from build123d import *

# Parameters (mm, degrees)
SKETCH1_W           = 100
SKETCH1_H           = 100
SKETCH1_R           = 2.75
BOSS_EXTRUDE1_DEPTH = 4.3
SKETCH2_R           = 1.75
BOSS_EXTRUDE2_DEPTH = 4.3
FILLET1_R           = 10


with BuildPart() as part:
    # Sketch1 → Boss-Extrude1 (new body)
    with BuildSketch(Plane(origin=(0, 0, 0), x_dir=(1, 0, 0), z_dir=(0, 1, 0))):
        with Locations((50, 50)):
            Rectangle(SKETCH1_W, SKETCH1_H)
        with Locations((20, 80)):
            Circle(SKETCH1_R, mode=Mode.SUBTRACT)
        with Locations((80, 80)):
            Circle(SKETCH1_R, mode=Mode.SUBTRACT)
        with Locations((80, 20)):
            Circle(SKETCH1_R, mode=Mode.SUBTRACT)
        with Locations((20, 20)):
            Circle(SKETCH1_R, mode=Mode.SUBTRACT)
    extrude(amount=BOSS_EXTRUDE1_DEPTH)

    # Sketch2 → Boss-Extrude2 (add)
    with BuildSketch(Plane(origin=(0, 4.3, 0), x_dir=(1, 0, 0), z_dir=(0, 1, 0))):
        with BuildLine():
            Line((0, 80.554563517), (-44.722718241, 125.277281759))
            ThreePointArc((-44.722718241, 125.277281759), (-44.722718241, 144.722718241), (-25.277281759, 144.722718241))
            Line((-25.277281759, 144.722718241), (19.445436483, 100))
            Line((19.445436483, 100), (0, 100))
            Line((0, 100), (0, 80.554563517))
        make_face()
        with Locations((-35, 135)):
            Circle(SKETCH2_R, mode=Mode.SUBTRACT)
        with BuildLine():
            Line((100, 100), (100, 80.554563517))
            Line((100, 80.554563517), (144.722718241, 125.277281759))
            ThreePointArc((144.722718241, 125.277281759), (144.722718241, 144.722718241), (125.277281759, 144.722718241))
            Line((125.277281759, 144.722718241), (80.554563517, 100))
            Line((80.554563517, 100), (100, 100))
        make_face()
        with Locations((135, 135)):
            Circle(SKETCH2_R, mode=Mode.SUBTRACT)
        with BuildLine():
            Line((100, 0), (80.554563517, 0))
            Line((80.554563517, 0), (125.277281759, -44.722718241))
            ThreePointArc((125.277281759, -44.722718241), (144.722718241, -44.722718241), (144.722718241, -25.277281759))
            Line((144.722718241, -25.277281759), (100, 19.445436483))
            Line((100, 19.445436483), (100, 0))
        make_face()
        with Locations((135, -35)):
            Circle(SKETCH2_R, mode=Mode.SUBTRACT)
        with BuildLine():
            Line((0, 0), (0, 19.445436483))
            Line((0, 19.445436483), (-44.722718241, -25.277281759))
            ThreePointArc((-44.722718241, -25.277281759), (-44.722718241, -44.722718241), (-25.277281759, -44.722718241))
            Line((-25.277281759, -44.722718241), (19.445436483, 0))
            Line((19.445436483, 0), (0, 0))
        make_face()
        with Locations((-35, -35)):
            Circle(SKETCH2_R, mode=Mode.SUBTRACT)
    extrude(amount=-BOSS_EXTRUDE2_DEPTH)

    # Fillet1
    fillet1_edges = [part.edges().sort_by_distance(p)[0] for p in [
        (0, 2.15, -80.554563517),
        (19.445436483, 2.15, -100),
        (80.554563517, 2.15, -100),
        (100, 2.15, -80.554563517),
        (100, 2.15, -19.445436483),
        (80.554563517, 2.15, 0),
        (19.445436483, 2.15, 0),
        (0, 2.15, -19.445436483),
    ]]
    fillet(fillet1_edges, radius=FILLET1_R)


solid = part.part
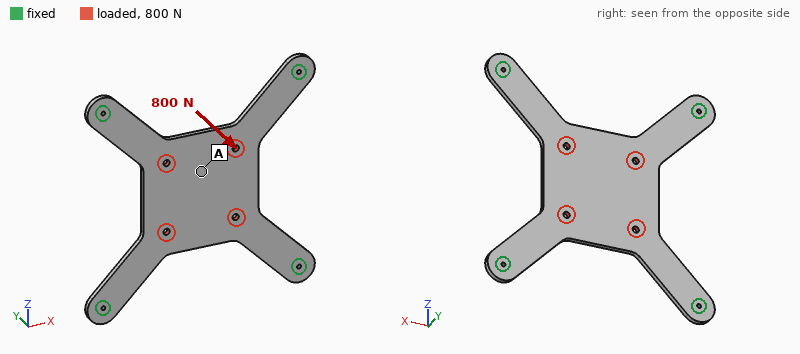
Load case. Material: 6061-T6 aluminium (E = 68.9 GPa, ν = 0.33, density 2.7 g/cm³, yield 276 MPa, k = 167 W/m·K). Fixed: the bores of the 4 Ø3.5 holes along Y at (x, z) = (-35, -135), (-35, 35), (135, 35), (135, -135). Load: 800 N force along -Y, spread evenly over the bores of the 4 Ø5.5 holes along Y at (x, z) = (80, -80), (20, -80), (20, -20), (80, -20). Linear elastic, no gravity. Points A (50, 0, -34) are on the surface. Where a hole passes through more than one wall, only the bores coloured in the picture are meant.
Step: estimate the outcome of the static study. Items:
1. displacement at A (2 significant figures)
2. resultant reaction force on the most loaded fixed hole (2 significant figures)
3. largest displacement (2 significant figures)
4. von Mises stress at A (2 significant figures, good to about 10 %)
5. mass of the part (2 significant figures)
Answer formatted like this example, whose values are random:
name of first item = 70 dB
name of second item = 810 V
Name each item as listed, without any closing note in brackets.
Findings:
displacement at A = 0.99 mm
resultant reaction force on the most loaded fixed hole = 200 N
largest displacement = 1.0 mm
von Mises stress at A = 29 MPa
mass of the part = 200 g
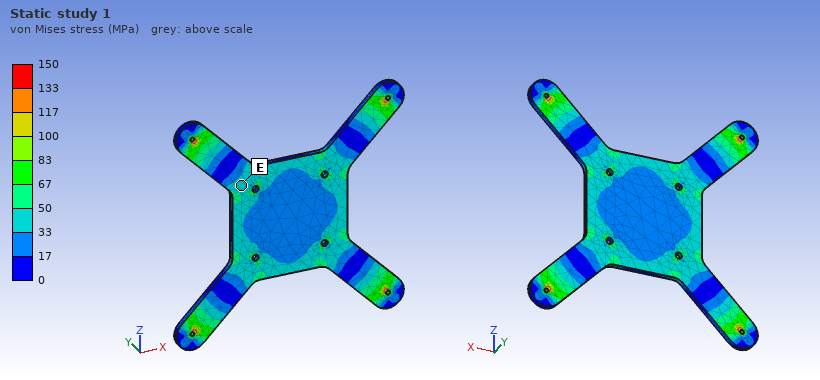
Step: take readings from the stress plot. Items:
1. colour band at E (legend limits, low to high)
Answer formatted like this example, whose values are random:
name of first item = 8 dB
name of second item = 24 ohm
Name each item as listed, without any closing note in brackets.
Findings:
colour band at E = 33 to 50 MPa
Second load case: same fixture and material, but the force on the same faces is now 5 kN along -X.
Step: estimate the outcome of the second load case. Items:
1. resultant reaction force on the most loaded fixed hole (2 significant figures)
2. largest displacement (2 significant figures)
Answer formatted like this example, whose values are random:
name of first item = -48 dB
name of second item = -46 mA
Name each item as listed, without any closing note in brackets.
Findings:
resultant reaction force on the most loaded fixed hole = 1.7 kN
largest displacement = 29 µm
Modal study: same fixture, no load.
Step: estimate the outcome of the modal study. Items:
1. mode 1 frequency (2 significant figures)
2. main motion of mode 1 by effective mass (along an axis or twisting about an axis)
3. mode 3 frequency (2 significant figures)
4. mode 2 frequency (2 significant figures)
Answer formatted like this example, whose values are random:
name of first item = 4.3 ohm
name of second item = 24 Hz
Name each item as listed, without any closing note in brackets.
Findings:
mode 1 frequency = 420 Hz
main motion of mode 1 by effective mass = along Y
mode 3 frequency = 980 Hz
mode 2 frequency = 980 Hz
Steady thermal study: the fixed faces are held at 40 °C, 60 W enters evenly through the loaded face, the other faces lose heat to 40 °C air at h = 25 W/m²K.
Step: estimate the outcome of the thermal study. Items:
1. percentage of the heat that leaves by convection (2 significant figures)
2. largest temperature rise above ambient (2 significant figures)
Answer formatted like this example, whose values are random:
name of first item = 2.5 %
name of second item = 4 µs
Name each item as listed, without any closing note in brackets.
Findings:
percentage of the heat that leaves by convection = 41 %
largest temperature rise above ambient = 42 K
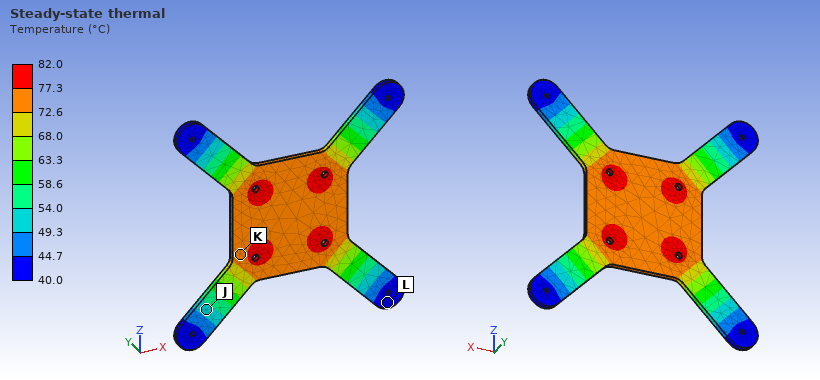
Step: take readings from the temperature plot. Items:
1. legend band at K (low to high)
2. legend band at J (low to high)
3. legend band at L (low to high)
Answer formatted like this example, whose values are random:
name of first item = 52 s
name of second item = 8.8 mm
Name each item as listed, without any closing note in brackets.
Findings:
legend band at K = 72.6 to 77.3 °C
legend band at J = 49.3 to 54.0 °C
legend band at L = 40.0 to 44.7 °C
